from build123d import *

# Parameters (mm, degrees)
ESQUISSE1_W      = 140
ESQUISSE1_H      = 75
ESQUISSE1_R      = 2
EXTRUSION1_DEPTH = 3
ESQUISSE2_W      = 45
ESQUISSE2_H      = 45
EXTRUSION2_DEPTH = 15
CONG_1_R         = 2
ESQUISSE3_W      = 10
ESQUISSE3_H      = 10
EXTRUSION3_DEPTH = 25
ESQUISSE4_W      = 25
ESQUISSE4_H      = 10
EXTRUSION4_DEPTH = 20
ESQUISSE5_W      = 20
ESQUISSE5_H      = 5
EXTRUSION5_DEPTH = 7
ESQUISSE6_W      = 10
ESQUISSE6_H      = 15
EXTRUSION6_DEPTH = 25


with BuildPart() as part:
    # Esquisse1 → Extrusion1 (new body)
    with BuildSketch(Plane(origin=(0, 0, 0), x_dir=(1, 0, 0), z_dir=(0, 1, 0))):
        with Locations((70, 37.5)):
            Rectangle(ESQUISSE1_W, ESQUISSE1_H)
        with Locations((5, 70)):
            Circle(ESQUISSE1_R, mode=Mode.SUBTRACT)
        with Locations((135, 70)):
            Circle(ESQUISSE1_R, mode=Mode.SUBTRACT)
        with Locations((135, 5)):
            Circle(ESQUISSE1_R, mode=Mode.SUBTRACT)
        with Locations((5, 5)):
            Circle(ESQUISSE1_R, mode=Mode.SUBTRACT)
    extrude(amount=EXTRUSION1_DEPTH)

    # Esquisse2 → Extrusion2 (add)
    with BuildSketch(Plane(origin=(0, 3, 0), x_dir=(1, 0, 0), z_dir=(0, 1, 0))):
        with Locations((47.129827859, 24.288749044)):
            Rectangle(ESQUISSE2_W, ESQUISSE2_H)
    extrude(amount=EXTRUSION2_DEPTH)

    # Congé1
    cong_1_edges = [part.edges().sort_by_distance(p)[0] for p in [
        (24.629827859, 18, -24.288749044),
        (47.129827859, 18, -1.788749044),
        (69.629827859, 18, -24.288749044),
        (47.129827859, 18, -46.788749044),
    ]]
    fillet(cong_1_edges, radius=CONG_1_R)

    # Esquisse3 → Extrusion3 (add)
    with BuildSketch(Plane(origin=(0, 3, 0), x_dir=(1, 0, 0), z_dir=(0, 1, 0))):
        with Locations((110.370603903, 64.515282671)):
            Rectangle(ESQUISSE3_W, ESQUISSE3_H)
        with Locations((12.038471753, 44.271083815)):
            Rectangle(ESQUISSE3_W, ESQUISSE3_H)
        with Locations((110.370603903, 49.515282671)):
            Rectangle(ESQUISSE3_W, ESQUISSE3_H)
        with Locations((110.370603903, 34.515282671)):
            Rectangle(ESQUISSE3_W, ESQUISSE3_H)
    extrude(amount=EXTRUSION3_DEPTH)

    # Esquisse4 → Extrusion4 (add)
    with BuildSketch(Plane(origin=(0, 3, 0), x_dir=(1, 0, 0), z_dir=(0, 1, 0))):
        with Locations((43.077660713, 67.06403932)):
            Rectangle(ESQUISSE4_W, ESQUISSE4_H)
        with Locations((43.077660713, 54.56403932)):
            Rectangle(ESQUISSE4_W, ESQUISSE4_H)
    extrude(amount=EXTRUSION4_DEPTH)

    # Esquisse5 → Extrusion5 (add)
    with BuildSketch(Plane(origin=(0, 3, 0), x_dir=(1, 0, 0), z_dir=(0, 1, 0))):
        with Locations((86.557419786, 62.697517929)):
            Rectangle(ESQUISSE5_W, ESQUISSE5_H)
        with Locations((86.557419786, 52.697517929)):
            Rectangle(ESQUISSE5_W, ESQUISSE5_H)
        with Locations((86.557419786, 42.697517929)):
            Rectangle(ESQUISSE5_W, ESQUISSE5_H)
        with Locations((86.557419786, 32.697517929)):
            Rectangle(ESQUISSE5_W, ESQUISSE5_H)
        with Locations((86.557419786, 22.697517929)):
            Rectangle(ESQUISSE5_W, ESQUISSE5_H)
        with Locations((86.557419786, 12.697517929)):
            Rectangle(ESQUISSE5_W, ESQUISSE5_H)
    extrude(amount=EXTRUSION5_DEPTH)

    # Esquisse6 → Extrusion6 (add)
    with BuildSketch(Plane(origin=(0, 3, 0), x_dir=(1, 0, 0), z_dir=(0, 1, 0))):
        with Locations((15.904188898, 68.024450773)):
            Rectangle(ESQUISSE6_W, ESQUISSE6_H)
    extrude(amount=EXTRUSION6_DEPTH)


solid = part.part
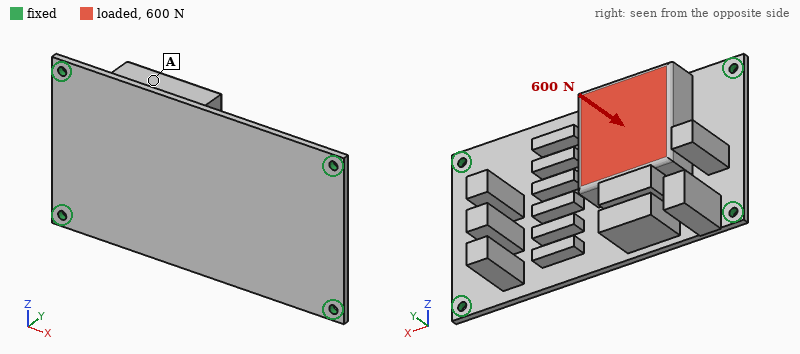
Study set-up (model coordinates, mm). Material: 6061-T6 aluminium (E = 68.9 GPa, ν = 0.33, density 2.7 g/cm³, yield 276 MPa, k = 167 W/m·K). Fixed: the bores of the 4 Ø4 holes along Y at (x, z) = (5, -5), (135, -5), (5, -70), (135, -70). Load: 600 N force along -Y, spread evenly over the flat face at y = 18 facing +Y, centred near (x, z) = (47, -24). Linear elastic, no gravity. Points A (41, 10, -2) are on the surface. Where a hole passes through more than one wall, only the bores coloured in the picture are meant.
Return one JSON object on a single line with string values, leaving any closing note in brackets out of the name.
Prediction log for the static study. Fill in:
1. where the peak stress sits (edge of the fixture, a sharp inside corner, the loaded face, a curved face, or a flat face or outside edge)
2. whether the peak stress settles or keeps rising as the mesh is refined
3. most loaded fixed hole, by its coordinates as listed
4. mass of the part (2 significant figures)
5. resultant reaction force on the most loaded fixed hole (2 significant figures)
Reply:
{"where the peak stress sits": "edge of the fixture", "whether the peak stress settles or keeps rising as the mesh is refined": "keeps rising", "most loaded fixed hole, by its coordinates as listed": "(5, -5)", "mass of the part": "240 g", "resultant reaction force on the most loaded fixed hole": "370 N"}
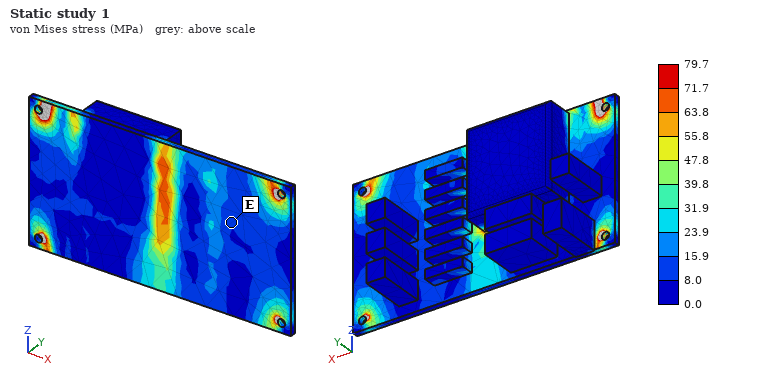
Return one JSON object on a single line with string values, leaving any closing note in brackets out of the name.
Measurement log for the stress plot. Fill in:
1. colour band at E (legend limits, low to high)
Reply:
{"colour band at E": "8.0 to 15.9 MPa"}
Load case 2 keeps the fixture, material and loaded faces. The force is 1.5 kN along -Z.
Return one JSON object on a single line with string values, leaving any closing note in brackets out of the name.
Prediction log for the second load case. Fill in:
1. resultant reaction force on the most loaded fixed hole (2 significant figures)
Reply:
{"resultant reaction force on the most loaded fixed hole": "840 N"}
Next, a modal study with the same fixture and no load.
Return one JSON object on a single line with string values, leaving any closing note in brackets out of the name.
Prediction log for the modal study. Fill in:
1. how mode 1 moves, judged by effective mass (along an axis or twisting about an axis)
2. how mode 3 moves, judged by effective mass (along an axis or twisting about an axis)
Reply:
{"how mode 1 moves, judged by effective mass": "along Y", "how mode 3 moves, judged by effective mass": "twisting about Z"}
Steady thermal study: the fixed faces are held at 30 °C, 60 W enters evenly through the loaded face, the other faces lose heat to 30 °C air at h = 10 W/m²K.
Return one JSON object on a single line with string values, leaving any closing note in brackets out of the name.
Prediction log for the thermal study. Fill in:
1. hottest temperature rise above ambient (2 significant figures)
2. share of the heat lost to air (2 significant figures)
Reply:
{"hottest temperature rise above ambient": "43 K", "share of the heat lost to air": "14 %"}
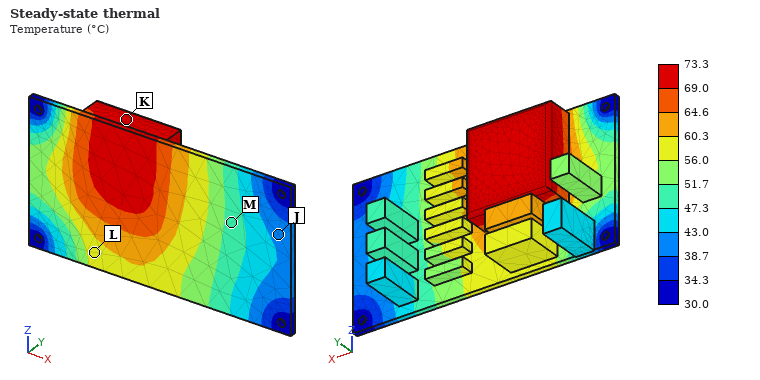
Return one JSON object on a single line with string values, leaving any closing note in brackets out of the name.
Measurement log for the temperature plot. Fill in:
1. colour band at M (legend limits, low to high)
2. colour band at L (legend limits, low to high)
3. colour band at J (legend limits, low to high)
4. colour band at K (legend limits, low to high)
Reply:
{"colour band at M": "47.3 to 51.7 °C", "colour band at L": "56.0 to 60.3 °C", "colour band at J": "38.7 to 43.0 °C", "colour band at K": "69.0 to 73.3 °C"}
